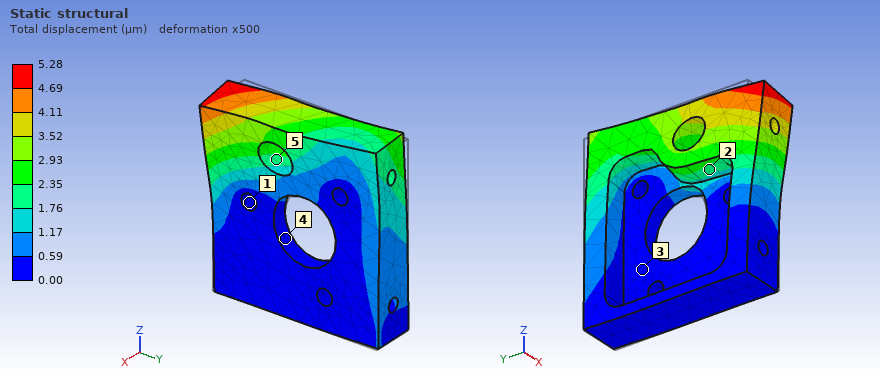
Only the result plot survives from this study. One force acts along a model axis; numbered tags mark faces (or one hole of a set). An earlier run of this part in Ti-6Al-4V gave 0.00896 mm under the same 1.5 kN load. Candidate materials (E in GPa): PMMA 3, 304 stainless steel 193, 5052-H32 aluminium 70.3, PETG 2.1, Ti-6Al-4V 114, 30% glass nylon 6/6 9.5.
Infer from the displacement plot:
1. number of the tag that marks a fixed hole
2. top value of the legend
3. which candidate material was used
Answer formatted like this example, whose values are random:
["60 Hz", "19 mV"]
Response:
["1", "5.28 µm", "304 stainless steel"]
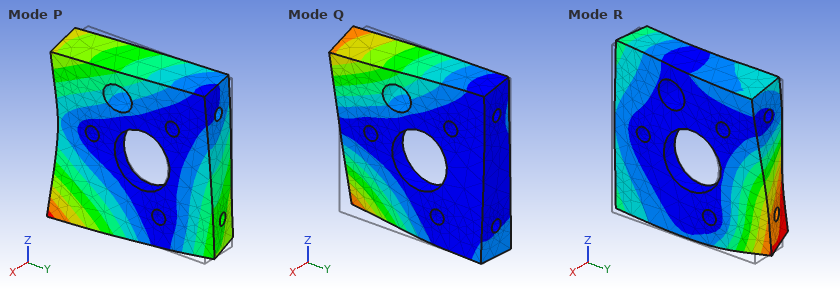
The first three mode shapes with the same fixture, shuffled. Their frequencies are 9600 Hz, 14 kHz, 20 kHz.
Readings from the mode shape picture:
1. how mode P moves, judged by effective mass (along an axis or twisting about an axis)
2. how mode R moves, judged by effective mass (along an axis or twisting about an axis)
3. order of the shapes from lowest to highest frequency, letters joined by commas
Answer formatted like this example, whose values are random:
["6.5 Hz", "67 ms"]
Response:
["along X", "along X", "Q, P, R"]
